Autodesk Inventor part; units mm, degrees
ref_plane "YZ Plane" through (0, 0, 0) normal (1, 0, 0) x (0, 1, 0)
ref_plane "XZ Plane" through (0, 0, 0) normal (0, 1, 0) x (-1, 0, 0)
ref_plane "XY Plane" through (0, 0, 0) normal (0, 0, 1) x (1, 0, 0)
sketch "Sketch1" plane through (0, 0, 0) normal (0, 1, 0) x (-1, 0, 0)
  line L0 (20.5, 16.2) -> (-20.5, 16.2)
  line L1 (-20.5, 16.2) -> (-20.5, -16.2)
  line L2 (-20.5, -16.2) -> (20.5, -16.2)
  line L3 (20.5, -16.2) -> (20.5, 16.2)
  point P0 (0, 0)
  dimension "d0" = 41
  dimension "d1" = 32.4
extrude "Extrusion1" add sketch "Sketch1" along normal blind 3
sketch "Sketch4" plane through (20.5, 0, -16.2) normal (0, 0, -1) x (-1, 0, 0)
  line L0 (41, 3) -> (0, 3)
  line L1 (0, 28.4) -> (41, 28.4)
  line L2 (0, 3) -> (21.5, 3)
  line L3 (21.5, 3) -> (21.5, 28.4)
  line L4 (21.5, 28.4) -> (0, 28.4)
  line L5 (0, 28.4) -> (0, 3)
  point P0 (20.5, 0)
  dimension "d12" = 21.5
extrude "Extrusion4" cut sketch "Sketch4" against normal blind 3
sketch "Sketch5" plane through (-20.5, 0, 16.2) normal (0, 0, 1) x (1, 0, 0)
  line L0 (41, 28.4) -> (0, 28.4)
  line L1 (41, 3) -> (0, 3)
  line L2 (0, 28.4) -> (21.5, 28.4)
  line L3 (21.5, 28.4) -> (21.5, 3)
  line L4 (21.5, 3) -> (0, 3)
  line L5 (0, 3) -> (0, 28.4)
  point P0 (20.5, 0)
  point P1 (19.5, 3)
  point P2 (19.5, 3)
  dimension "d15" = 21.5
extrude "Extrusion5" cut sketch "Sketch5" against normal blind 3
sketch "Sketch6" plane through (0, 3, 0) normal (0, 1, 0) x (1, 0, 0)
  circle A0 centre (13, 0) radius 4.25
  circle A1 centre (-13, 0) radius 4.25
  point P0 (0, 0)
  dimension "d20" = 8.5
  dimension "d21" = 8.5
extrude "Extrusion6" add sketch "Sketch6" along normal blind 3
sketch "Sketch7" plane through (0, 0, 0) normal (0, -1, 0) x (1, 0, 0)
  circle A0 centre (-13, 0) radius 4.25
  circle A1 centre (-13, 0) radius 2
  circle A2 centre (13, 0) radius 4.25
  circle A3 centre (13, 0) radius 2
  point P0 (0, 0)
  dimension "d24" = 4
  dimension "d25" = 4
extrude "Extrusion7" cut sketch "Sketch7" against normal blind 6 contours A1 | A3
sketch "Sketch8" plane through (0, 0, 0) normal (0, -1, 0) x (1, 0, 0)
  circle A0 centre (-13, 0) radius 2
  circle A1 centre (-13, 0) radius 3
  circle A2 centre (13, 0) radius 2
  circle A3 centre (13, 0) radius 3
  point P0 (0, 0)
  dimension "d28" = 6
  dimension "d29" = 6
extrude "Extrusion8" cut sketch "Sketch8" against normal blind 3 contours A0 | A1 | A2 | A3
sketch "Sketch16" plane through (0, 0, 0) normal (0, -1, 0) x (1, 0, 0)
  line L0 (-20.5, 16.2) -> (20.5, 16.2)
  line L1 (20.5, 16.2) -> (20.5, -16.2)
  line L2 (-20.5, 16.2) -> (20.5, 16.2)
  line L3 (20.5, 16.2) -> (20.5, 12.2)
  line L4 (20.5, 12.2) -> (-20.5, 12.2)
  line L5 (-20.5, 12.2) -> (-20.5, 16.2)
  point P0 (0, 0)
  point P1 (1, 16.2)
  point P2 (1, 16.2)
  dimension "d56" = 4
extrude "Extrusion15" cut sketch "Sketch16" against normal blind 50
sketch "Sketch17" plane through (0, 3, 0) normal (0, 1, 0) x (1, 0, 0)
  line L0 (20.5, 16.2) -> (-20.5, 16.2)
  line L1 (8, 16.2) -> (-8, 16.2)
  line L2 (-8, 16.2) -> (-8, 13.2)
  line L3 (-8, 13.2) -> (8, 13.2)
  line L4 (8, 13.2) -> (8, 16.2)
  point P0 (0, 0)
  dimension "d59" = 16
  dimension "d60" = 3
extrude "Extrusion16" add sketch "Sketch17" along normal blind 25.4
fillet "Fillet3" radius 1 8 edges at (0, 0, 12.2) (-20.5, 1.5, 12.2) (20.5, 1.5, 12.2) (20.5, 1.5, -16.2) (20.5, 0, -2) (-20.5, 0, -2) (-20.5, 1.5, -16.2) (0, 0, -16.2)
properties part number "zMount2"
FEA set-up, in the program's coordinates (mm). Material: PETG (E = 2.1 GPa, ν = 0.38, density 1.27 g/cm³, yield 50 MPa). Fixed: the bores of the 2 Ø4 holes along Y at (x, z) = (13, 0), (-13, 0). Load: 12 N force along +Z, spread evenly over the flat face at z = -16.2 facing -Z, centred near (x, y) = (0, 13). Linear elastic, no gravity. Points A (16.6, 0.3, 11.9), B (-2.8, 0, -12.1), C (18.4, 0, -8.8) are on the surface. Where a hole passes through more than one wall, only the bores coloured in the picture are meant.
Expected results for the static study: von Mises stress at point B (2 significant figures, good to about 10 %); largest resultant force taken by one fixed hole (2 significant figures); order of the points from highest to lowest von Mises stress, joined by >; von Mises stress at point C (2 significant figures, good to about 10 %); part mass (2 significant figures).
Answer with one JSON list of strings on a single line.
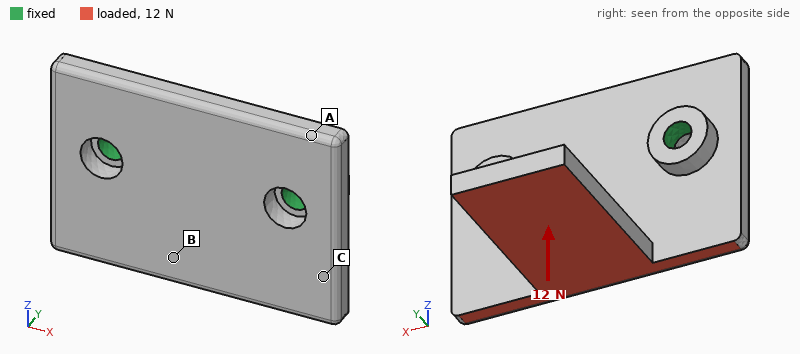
["3.7 MPa", "6.1 N", "B > C > A", "1.8 MPa", "6.1 g"]
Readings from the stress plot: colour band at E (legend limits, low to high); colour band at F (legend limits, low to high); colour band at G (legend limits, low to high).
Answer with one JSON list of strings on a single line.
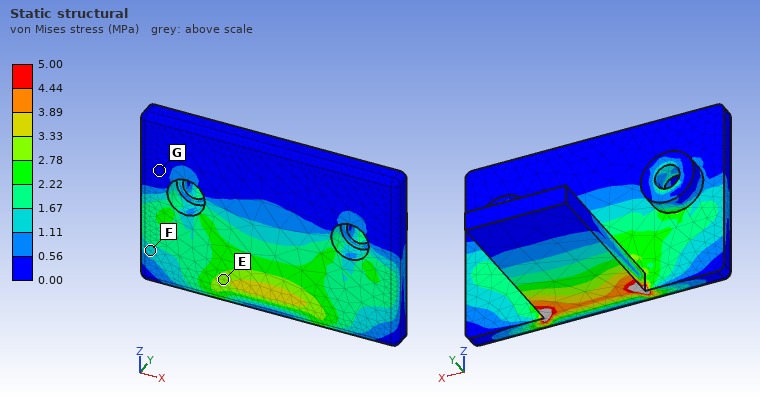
["2.78 to 3.33 MPa", "1.11 to 1.67 MPa", "0.00 to 0.56 MPa"]
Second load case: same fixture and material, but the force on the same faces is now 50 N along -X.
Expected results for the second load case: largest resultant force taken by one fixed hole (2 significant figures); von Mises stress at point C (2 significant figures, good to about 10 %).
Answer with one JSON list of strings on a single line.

["41 N", "2.8 MPa"]
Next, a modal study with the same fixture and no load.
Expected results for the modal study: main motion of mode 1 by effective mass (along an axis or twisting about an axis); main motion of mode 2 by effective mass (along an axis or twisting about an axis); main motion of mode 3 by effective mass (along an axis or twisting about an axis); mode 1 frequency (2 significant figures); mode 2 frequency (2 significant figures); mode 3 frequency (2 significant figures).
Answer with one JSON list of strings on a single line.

["along Z", "along X", "along Y", "590 Hz", "1200 Hz", "1500 Hz"]
